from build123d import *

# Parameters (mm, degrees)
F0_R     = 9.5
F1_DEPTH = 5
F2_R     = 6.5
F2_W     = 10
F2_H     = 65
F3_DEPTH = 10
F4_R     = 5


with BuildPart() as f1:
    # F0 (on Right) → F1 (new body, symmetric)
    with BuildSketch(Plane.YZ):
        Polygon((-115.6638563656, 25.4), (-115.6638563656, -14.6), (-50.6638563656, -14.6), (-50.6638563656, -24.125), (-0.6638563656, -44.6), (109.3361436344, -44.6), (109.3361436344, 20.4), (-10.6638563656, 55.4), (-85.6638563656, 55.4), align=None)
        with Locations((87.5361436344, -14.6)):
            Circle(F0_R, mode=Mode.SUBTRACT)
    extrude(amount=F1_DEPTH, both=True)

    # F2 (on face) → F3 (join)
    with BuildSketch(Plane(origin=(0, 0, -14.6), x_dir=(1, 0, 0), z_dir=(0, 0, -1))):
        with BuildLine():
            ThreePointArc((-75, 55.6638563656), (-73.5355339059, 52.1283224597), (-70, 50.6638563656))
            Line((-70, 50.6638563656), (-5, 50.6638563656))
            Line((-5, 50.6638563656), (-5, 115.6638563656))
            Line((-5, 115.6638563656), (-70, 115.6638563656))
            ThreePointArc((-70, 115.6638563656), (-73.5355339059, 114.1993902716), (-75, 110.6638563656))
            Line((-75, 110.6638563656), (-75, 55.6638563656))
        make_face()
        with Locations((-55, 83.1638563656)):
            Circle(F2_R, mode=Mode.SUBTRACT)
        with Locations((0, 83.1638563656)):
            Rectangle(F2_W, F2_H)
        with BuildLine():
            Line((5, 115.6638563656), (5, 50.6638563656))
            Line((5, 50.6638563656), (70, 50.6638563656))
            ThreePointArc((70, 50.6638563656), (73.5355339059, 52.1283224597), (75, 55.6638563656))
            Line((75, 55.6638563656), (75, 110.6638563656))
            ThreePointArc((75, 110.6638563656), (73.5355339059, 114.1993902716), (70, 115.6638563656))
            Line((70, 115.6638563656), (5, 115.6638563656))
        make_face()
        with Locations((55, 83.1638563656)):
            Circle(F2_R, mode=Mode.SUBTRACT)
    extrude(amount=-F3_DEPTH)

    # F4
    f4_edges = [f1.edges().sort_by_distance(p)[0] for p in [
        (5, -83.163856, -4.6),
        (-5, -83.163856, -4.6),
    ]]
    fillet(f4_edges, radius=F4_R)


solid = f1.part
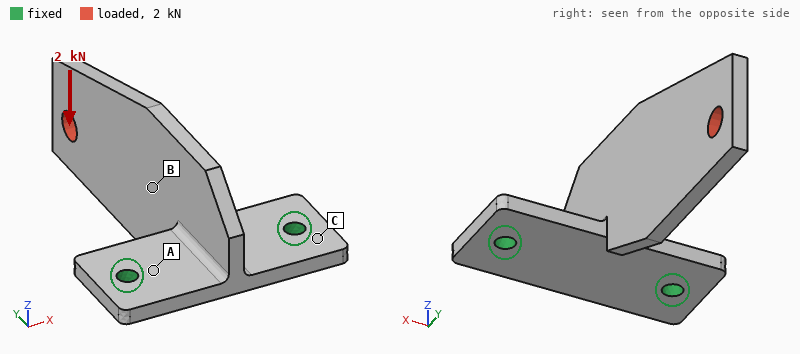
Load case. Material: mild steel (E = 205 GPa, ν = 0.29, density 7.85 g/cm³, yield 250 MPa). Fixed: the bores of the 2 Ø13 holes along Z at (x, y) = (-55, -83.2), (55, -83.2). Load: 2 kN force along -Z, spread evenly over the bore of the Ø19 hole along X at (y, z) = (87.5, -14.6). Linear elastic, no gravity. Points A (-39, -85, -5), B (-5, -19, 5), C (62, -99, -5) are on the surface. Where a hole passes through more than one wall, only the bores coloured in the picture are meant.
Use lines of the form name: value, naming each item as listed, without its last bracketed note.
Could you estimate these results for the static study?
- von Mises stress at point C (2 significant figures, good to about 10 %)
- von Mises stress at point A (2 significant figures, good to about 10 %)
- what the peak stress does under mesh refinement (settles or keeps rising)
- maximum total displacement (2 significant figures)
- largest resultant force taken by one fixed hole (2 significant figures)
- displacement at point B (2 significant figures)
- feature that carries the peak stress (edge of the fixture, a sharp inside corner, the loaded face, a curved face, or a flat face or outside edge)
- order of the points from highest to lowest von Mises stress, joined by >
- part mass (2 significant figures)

von Mises stress at point C: 69 MPa
von Mises stress at point A: 130 MPa
what the peak stress does under mesh refinement: keeps rising
maximum total displacement: 0.87 mm
largest resultant force taken by one fixed hole: 1.2 kN
displacement at point B: 0.29 mm
feature that carries the peak stress: edge of the fixture
order of the points from highest to lowest von Mises stress, joined by >: A > C > B
part mass: 2.0 kg
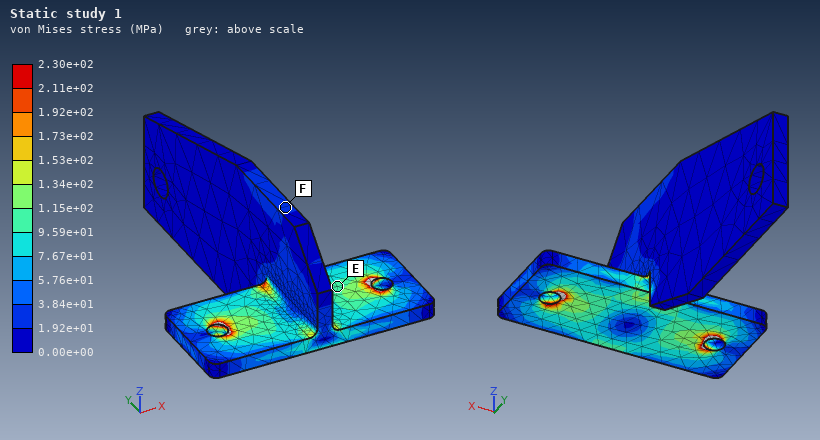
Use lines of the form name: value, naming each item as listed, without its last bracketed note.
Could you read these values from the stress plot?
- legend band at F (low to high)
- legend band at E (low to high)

legend band at F: 1.92e+01 to 3.84e+01 MPa
legend band at E: 9.59e+01 to 1.15e+02 MPa
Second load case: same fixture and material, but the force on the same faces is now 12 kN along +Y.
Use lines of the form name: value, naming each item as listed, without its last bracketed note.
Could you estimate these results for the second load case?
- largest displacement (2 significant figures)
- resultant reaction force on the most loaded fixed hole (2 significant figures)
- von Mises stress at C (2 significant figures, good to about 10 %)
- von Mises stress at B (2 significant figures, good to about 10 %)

largest displacement: 0.21 mm
resultant reaction force on the most loaded fixed hole: 6.1 kN
von Mises stress at C: 16 MPa
von Mises stress at B: 23 MPa
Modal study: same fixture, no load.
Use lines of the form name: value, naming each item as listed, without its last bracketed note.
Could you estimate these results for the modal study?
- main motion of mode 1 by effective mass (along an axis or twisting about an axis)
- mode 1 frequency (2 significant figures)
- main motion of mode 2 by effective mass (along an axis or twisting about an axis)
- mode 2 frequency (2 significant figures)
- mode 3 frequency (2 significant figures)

main motion of mode 1 by effective mass: along X
mode 1 frequency: 290 Hz
main motion of mode 2 by effective mass: along Z
mode 2 frequency: 360 Hz
mode 3 frequency: 910 Hz
